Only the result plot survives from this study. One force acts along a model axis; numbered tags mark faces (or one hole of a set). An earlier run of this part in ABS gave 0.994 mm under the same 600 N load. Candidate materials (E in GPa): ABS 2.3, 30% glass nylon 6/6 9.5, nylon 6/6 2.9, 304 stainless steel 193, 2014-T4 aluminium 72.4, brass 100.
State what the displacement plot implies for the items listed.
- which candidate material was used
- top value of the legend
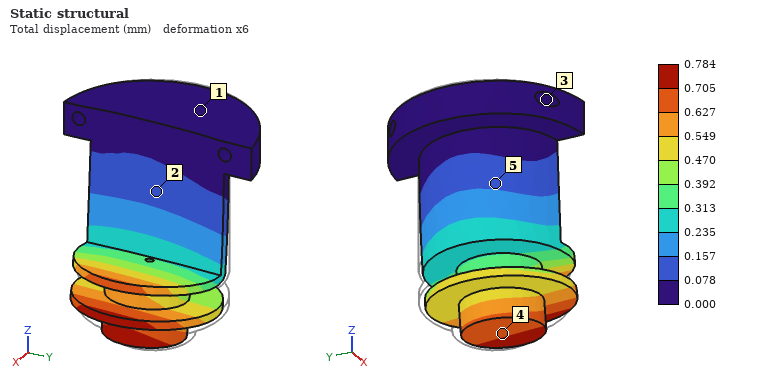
nylon 6/6
0.784 mm
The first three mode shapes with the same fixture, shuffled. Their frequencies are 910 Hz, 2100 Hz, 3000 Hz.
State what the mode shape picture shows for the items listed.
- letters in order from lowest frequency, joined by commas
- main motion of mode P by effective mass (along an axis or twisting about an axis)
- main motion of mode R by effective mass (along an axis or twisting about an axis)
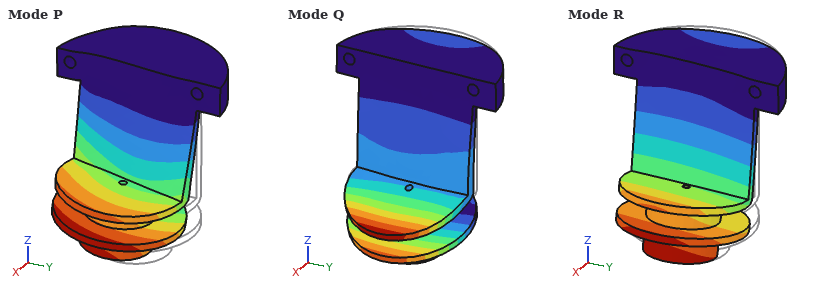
R, P, Q
along Y
along X
